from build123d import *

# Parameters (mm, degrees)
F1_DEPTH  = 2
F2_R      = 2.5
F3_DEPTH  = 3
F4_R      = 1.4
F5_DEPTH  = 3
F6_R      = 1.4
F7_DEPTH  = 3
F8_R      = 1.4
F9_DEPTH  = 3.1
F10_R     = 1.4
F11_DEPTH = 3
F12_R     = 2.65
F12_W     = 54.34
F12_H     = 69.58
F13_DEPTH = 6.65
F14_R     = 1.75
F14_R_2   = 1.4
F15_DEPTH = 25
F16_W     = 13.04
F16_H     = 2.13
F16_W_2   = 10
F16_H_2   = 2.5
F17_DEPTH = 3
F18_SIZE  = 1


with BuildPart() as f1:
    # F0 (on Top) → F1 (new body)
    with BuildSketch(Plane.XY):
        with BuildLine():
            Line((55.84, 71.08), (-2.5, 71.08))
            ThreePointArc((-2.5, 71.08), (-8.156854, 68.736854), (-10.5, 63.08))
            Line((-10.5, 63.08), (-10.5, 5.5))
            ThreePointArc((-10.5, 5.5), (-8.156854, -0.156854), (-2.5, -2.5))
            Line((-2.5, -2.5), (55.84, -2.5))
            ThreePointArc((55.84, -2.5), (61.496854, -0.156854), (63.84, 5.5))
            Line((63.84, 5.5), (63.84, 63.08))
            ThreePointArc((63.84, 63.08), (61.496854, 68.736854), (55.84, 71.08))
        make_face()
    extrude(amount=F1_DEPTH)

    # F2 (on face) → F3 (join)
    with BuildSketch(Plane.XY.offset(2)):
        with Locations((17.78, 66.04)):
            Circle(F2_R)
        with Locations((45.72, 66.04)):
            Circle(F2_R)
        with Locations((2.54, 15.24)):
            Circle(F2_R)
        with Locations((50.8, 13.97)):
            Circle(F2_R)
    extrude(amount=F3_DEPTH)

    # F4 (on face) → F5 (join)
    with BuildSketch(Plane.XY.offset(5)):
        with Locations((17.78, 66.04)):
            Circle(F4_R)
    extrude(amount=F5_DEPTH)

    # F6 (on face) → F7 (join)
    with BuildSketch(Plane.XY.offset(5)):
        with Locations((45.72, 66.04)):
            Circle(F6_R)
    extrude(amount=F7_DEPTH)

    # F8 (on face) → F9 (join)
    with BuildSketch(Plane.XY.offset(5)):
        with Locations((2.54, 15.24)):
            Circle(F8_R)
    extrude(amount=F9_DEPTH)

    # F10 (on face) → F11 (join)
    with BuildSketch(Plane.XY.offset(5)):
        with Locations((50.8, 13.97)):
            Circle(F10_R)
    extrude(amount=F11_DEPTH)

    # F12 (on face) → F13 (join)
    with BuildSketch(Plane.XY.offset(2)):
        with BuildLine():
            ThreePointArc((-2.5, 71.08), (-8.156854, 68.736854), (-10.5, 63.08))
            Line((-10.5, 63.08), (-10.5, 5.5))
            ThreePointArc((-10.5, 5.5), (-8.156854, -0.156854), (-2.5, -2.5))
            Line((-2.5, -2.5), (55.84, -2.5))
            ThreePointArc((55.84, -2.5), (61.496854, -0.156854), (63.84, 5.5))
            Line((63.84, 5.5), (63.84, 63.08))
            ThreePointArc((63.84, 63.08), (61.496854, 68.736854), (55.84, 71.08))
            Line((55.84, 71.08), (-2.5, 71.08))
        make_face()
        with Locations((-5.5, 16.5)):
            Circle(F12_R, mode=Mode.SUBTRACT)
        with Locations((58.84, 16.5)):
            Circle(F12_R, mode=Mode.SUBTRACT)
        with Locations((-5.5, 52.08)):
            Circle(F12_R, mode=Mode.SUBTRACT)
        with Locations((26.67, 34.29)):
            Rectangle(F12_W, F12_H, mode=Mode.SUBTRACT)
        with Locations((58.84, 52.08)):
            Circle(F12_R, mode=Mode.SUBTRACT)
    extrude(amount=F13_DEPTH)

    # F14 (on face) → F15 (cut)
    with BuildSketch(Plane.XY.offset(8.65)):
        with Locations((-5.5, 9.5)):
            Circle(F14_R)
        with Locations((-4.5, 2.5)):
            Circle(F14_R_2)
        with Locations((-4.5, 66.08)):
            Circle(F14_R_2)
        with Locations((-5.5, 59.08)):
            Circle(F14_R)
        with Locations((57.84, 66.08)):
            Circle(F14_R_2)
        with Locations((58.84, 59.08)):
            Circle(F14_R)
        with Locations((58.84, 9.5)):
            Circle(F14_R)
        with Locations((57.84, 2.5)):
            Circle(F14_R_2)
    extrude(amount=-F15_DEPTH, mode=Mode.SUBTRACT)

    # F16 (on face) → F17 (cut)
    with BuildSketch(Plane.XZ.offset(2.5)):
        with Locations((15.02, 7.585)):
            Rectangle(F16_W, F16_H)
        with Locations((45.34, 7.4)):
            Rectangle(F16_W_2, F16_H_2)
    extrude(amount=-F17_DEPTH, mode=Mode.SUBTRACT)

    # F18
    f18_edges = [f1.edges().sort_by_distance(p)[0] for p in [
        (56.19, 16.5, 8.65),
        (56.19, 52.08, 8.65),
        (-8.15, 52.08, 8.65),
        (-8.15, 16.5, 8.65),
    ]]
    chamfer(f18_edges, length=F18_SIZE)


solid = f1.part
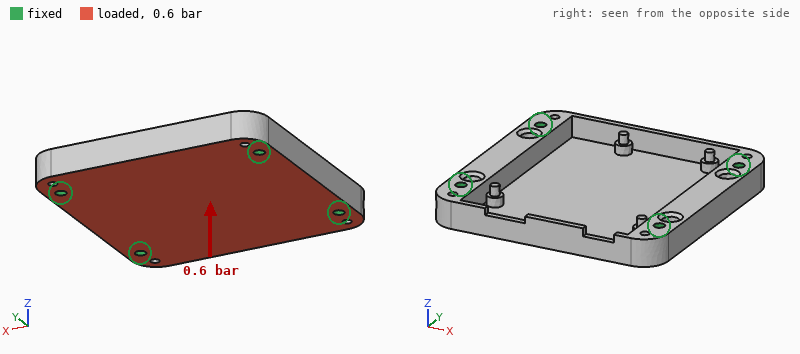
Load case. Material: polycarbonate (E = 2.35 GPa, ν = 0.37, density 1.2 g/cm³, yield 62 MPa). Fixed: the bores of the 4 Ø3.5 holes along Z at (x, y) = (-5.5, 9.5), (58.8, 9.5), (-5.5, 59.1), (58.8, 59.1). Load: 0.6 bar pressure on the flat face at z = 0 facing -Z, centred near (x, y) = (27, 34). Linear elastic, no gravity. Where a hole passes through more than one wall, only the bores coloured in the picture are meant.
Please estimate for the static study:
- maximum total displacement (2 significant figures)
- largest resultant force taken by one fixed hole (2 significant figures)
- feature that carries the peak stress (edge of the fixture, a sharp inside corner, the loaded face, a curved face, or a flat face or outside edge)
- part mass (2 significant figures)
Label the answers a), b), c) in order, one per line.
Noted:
a) 0.83 mm
b) 90 N
c) the loaded face
d) 25 g
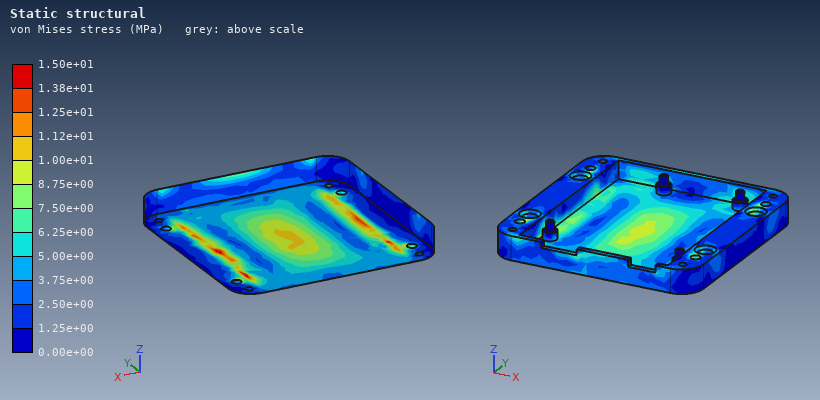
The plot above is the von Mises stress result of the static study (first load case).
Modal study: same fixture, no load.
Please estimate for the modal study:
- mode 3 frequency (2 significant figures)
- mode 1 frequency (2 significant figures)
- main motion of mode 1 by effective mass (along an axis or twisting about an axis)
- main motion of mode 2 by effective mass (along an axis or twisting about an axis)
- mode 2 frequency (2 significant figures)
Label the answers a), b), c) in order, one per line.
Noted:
a) 2100 Hz
b) 1100 Hz
c) along Z
d) twisting about X
e) 1600 Hz
